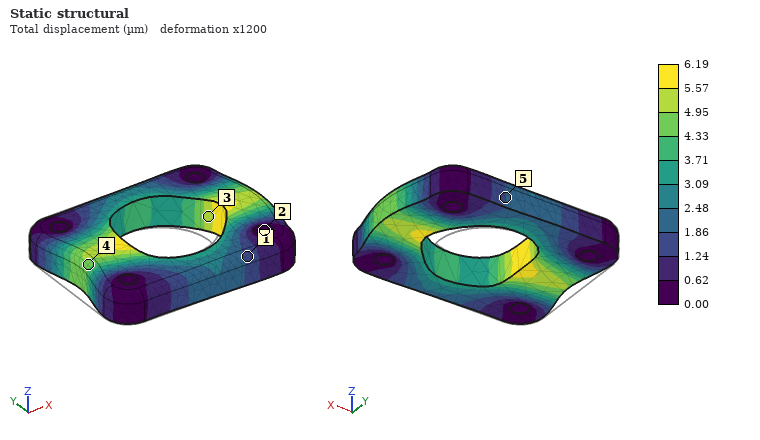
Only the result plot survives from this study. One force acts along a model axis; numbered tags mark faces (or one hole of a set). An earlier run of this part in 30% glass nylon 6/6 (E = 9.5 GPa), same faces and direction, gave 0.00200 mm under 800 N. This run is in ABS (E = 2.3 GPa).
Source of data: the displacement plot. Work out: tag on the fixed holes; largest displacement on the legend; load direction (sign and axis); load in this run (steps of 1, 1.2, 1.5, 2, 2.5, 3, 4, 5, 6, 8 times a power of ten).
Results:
2
6.19 µm
+X
600 N
